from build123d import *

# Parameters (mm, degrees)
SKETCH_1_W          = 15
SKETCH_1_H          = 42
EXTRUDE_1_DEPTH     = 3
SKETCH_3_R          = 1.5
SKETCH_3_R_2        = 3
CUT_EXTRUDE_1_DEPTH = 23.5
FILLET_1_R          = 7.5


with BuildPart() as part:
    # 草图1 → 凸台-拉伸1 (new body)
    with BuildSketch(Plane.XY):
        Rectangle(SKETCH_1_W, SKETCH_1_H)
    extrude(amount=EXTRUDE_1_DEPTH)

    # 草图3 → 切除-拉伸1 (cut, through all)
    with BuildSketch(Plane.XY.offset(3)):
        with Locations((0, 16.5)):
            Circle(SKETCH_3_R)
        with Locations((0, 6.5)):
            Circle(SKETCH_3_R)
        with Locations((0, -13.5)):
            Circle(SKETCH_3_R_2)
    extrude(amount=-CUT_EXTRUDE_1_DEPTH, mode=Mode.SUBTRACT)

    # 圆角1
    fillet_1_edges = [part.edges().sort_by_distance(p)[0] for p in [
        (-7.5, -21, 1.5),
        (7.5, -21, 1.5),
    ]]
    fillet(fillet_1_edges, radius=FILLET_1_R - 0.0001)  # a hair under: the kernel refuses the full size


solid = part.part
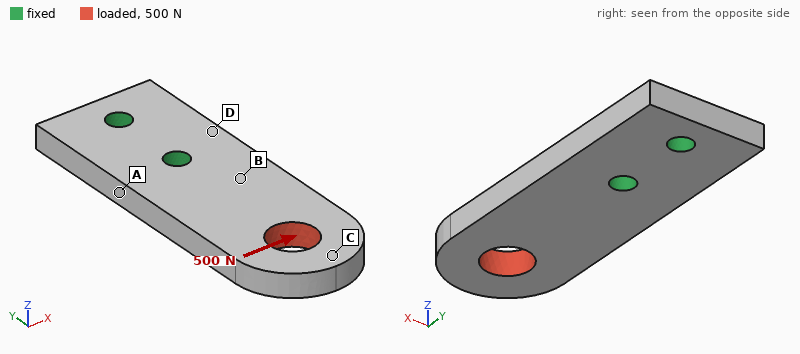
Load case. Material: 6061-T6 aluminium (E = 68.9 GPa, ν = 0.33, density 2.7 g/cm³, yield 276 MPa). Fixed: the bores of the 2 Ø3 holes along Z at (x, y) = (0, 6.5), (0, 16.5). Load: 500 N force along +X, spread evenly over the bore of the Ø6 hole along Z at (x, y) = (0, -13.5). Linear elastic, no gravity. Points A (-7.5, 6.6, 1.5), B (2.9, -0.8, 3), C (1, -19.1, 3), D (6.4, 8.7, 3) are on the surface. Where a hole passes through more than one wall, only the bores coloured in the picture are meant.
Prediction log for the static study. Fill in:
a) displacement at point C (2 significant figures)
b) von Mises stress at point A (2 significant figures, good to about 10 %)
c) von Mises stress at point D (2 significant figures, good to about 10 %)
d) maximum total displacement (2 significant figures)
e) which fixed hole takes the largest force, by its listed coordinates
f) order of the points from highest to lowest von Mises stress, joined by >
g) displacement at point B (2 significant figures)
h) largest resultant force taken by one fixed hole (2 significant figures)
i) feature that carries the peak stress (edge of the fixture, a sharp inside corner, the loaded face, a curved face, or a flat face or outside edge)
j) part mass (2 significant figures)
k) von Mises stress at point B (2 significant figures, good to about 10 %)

76 µm
81 MPa
53 MPa
81 µm
(0, 6.5)
A > D > B > C
17 µm
1.2 kN
edge of the fixture
4.6 g
32 MPa
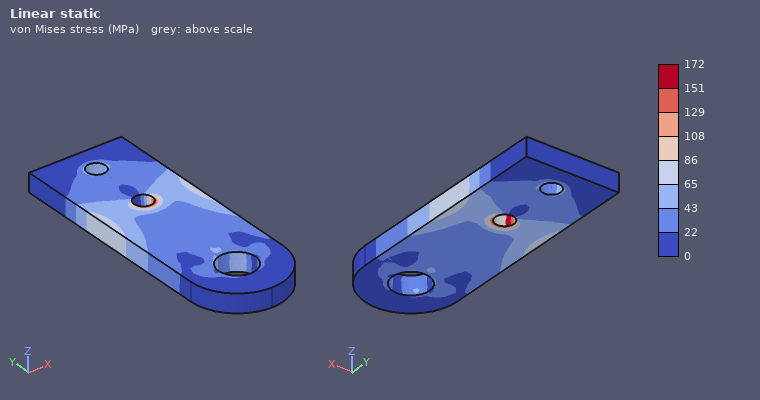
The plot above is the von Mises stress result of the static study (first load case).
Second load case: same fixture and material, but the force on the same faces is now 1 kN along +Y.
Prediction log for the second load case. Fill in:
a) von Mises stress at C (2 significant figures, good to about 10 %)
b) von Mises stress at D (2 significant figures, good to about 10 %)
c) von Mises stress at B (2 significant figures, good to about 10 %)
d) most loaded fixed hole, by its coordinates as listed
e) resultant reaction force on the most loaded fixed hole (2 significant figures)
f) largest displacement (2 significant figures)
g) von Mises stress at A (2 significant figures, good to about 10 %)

17 MPa
11 MPa
24 MPa
(0, 6.5)
800 N
11 µm
13 MPa
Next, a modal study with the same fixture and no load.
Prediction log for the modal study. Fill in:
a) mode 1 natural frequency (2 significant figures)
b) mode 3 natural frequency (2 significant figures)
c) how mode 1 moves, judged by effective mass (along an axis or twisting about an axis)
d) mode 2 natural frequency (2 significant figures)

3900 Hz
12 kHz
along Z
12 kHz
